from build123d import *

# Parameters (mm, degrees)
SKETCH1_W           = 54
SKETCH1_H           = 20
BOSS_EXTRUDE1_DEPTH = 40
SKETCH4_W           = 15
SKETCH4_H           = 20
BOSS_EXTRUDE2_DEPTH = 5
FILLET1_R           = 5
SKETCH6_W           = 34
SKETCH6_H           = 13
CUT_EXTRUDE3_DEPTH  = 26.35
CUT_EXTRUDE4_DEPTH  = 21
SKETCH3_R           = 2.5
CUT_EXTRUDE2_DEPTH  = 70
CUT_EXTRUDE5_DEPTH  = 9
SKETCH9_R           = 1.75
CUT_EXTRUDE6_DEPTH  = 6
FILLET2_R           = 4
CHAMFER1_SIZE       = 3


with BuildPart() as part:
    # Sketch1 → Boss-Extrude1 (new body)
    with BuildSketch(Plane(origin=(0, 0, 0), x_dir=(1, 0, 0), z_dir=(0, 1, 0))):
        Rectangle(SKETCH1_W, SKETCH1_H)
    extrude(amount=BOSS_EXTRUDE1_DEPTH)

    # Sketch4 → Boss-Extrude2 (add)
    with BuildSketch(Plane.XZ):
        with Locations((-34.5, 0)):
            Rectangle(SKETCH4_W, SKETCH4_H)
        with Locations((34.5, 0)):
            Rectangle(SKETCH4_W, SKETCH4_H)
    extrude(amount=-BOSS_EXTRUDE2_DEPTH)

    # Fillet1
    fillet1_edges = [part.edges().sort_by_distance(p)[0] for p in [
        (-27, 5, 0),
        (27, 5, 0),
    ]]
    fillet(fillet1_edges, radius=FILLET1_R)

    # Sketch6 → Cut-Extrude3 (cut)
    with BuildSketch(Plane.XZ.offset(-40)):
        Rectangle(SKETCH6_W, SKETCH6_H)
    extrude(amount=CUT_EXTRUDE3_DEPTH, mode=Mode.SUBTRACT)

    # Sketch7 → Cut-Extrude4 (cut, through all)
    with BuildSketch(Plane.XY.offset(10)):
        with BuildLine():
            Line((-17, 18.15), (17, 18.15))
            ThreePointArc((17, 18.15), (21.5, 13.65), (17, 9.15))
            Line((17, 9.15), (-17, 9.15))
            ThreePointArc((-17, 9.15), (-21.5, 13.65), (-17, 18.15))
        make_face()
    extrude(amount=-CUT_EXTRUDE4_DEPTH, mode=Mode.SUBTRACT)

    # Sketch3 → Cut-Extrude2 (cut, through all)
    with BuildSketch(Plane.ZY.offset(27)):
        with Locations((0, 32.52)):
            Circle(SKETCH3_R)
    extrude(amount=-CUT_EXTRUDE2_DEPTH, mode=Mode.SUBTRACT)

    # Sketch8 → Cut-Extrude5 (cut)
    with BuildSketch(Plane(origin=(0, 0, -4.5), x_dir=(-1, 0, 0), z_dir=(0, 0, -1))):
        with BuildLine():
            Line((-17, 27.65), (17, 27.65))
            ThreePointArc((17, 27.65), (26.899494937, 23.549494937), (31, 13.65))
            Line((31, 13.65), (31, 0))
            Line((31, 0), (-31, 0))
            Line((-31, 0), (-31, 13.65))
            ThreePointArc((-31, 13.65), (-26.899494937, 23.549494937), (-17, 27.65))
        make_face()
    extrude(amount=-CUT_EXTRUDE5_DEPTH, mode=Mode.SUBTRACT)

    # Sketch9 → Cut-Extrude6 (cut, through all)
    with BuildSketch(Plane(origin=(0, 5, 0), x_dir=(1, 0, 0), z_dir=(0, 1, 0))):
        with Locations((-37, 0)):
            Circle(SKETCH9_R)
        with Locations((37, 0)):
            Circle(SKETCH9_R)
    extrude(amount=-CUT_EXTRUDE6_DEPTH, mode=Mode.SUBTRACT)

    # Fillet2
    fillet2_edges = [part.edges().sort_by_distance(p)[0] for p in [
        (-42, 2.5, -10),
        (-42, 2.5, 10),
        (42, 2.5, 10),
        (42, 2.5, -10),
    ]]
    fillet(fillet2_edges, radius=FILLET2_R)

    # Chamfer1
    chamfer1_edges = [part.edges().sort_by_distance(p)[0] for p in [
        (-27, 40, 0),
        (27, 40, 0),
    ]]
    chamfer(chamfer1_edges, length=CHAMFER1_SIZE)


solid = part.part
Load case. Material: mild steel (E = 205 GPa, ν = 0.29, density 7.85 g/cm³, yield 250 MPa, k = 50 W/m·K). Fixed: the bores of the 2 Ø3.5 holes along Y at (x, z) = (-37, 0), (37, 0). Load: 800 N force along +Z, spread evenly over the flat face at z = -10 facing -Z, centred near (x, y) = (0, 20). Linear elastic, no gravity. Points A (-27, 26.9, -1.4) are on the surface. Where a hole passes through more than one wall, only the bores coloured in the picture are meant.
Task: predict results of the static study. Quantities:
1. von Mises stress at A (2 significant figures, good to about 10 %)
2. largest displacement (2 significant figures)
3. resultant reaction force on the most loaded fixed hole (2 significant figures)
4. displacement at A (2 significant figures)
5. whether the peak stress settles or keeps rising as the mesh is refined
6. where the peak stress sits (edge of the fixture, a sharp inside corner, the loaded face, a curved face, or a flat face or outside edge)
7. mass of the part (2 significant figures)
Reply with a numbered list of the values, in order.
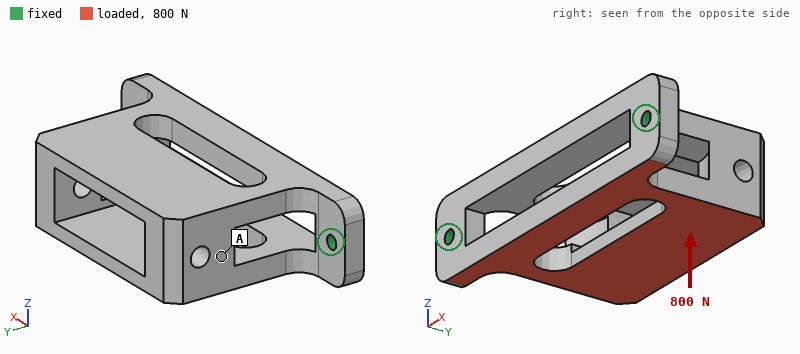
1. 14 MPa
2. 76 µm
3. 410 N
4. 51 µm
5. keeps rising
6. edge of the fixture
7. 170 g
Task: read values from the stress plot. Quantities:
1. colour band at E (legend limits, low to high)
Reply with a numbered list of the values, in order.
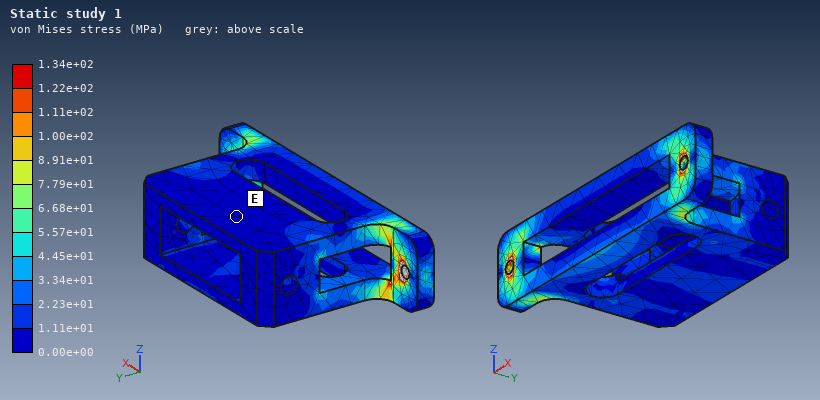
1. 0.00e+00 to 1.11e+01 MPa
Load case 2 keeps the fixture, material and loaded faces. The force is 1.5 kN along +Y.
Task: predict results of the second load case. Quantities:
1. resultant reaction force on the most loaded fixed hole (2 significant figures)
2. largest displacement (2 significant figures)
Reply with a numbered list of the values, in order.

1. 870 N
2. 65 µm
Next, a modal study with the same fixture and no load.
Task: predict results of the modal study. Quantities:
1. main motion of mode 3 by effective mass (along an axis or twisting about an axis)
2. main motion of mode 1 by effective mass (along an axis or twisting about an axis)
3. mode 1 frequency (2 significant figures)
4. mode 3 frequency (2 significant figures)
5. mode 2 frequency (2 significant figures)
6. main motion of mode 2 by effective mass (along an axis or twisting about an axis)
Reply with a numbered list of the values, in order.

1. along Y
2. along Z
3. 1500 Hz
4. 5300 Hz
5. 4200 Hz
6. twisting about Y
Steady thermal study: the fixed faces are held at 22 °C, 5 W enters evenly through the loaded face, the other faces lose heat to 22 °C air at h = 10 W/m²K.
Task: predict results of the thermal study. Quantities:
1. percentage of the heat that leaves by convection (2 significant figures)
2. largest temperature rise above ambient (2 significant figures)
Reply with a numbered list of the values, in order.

1. 21 %
2. 18 K
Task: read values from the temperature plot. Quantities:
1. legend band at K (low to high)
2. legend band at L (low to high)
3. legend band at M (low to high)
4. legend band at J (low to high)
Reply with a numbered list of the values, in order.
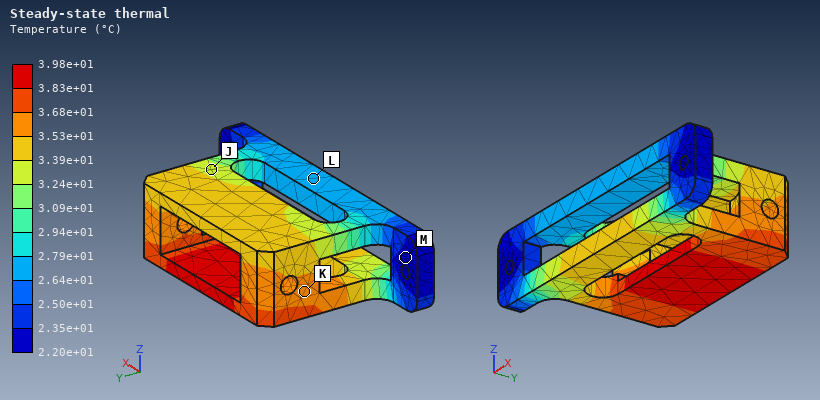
1. 3.53e+01 to 3.68e+01 °C
2. 2.64e+01 to 2.79e+01 °C
3. 2.20e+01 to 2.35e+01 °C
4. 3.24e+01 to 3.39e+01 °C
